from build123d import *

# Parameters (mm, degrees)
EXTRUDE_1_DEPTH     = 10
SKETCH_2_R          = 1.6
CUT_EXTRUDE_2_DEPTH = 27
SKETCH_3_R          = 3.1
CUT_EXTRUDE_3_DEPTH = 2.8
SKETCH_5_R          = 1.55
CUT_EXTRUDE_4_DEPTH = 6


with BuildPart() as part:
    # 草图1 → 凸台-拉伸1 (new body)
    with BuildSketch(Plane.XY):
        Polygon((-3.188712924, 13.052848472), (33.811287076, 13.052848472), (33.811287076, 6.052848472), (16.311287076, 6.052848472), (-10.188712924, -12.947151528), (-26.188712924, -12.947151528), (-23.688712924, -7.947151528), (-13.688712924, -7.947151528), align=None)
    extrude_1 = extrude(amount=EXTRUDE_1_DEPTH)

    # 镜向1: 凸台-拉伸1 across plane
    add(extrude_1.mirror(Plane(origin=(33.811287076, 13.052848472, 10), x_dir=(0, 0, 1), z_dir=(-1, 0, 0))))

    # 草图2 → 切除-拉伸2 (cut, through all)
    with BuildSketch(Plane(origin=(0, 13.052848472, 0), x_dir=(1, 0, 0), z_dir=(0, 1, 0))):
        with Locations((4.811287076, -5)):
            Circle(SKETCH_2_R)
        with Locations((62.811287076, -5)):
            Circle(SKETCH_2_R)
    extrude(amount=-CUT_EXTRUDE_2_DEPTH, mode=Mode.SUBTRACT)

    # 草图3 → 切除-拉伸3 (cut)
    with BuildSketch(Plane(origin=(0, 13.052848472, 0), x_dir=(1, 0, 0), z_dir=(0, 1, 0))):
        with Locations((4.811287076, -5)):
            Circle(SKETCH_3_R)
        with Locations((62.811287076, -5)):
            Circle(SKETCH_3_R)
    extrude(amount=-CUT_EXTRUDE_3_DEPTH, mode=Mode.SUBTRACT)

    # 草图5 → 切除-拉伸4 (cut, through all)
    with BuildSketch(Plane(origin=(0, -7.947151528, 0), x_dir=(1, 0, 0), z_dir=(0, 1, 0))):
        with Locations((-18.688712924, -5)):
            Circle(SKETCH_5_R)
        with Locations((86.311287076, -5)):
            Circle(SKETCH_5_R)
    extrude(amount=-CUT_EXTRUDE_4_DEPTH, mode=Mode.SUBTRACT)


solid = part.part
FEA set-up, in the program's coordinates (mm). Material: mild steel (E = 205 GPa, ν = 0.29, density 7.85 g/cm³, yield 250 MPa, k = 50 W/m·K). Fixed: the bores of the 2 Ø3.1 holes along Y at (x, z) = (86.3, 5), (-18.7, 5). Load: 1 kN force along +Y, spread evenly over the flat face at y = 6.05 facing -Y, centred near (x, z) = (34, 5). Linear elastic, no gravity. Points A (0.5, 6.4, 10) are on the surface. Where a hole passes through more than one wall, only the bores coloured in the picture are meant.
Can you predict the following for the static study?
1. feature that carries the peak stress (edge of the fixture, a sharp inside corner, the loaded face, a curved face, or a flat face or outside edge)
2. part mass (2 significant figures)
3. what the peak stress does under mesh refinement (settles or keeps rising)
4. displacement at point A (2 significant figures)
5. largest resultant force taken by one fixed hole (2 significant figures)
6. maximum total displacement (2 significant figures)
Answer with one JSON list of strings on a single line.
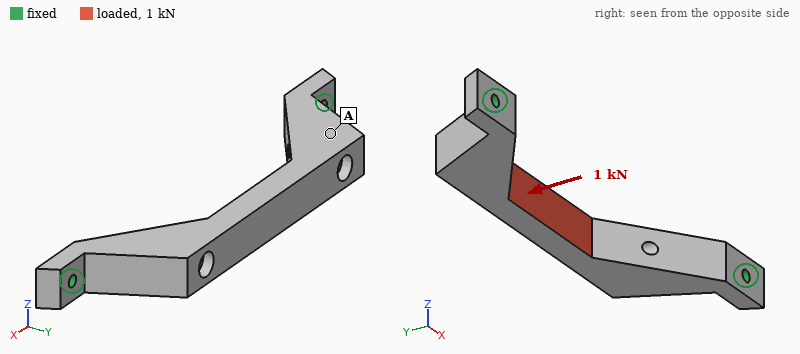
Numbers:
["edge of the fixture", "90 g", "keeps rising", "3.3 µm", "990 N", "15 µm"]
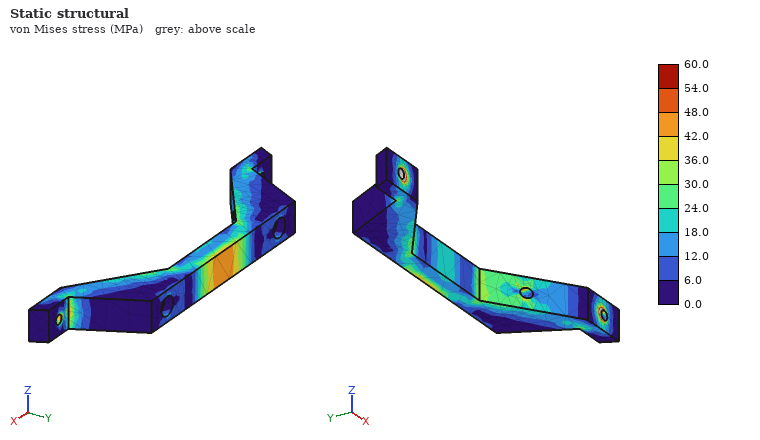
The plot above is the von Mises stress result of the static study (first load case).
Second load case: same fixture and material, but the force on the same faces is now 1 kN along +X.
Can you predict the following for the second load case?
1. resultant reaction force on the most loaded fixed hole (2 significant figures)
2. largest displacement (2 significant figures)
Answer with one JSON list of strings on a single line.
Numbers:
["520 N", "13 µm"]
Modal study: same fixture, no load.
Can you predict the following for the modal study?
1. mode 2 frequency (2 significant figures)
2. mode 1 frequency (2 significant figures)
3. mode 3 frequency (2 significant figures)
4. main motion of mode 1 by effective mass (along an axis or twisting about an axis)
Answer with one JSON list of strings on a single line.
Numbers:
["5600 Hz", "2200 Hz", "5800 Hz", "along Z"]
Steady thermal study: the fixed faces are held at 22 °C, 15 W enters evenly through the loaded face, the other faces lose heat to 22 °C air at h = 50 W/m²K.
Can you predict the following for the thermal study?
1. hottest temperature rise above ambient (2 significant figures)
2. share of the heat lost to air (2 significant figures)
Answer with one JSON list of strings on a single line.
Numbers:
["63 K", "47 %"]
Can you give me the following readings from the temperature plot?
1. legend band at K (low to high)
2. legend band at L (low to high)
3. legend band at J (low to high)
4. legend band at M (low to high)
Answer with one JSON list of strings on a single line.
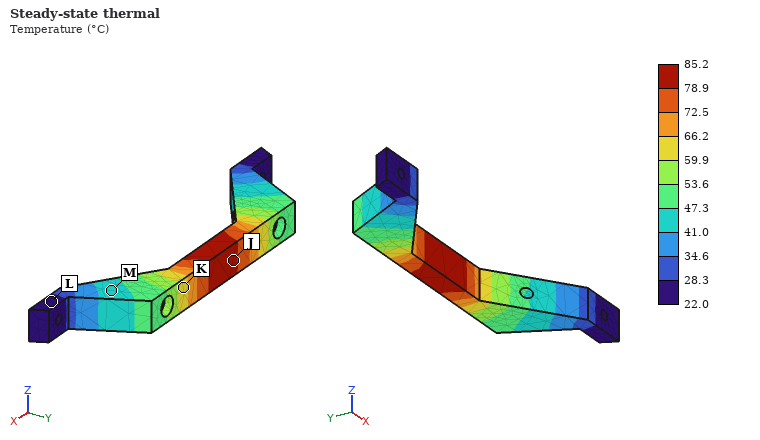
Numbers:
["59.9 to 66.2 °C", "22.0 to 28.3 °C", "78.9 to 85.2 °C", "41.0 to 47.3 °C"]
